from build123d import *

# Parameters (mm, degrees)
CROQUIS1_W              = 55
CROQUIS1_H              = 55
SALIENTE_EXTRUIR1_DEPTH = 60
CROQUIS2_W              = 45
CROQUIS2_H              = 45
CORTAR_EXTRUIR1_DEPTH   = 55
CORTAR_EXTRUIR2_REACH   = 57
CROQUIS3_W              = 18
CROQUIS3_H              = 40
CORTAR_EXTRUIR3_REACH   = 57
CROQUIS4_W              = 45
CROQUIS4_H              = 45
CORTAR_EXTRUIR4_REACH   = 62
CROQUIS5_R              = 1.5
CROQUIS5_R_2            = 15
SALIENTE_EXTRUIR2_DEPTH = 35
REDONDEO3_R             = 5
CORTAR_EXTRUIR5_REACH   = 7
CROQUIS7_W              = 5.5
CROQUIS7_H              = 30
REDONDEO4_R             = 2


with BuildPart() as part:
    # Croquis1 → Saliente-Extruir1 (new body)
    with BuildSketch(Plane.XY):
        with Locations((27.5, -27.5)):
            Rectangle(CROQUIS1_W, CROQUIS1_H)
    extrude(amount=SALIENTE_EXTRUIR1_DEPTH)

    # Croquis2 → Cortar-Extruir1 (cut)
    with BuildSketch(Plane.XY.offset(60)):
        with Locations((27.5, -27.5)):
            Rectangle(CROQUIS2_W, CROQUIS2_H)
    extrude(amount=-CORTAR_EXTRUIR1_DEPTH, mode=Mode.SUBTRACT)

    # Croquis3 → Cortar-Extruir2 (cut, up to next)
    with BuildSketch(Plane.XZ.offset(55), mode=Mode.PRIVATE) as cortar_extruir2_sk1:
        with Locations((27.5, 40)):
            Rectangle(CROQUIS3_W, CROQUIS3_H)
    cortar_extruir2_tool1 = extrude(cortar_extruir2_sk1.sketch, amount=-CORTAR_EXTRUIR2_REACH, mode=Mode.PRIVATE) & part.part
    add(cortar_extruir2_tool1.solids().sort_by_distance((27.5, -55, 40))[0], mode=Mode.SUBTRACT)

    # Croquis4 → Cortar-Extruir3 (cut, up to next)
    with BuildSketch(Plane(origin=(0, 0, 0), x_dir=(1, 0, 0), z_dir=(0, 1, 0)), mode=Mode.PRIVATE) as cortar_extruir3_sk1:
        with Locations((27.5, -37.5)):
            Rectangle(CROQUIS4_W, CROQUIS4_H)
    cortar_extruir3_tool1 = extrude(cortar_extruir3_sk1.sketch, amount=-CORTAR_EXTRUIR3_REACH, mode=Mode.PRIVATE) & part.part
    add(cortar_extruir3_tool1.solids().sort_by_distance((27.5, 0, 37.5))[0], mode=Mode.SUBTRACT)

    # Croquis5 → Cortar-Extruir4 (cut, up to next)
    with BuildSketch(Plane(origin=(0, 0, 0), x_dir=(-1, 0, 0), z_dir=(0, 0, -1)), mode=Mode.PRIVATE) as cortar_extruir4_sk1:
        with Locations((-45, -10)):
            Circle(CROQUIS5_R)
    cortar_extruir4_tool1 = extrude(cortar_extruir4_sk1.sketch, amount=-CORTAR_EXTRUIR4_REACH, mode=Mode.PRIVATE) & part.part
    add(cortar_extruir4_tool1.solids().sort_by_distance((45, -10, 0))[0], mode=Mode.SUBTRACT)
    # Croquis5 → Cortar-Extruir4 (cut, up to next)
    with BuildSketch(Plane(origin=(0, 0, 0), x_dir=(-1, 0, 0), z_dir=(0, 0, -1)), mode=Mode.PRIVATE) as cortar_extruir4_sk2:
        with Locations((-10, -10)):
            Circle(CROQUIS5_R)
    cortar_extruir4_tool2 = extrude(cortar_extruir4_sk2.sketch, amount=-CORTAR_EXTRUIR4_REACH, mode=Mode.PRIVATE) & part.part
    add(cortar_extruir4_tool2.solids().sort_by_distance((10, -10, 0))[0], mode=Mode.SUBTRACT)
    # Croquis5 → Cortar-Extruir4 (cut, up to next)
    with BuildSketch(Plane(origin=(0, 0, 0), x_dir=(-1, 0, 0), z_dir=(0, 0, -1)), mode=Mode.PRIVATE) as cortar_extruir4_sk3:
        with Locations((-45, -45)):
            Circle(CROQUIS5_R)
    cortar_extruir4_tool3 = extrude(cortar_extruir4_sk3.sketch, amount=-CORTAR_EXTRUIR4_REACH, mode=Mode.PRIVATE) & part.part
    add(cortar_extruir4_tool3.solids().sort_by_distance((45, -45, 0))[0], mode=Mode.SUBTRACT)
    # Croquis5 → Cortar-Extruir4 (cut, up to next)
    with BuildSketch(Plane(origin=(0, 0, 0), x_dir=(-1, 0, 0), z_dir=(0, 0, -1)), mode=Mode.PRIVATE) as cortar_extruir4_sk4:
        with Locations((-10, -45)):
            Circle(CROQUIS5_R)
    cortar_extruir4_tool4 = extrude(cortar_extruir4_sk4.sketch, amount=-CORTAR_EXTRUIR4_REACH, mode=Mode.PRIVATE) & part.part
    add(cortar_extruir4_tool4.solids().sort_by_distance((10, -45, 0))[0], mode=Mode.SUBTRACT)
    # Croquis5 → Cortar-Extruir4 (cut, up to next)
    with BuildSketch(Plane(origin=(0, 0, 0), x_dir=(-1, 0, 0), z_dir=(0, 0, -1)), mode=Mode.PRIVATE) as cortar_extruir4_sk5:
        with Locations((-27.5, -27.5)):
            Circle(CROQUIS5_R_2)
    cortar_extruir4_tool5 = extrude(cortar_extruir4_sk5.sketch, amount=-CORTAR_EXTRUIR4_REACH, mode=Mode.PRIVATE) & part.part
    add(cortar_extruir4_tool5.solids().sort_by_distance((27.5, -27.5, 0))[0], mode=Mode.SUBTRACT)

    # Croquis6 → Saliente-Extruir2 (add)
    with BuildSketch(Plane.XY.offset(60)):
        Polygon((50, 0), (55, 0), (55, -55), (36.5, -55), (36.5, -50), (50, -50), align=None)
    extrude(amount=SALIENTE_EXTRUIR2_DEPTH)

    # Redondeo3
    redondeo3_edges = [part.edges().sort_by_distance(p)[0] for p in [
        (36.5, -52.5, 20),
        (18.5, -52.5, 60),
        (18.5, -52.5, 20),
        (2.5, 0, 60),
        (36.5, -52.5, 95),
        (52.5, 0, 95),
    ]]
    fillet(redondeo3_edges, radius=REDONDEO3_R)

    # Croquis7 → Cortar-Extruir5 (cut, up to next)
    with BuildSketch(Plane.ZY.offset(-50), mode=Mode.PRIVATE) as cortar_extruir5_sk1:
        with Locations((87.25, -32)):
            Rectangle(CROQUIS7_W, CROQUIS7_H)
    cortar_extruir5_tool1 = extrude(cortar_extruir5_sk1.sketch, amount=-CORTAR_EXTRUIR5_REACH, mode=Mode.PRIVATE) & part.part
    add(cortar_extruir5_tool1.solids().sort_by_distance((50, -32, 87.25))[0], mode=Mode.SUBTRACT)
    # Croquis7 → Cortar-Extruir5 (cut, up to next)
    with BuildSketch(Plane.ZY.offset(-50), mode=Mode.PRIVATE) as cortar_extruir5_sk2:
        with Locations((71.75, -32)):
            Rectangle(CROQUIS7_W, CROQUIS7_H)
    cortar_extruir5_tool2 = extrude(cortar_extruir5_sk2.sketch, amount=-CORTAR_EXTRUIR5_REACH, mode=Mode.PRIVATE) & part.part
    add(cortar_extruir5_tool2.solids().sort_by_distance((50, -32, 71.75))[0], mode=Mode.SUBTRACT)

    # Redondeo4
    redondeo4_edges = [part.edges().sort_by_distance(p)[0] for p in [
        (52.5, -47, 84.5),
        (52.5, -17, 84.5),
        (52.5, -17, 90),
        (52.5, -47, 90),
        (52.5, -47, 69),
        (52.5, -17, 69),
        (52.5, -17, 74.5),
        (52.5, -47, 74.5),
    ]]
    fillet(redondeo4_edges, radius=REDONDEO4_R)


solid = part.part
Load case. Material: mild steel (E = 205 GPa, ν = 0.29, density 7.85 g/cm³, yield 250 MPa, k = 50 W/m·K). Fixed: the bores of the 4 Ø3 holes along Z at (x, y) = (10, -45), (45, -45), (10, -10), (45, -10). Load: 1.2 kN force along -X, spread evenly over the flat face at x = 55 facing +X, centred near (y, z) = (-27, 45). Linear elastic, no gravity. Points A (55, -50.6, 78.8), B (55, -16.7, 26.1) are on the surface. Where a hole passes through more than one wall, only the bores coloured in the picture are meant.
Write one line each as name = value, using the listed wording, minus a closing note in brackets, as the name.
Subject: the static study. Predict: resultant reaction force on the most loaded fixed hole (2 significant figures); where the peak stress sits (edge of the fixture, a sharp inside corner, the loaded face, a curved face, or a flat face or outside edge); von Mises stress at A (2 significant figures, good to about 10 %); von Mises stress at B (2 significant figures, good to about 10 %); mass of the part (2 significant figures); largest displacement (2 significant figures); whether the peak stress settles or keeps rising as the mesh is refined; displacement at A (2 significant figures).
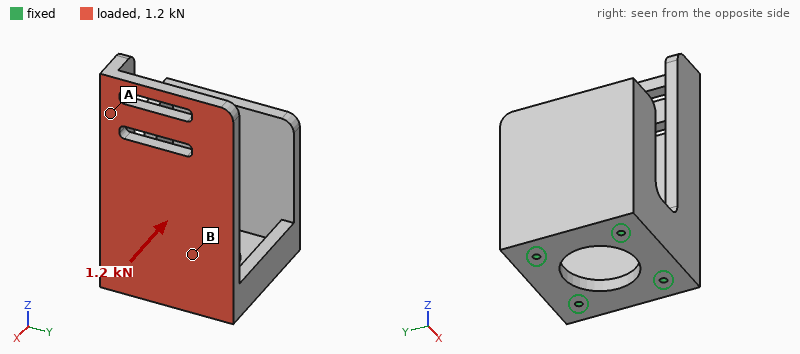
resultant reaction force on the most loaded fixed hole = 1.2 kN
where the peak stress sits = edge of the fixture
von Mises stress at A = 21 MPa
von Mises stress at B = 45 MPa
mass of the part = 490 g
largest displacement = 0.27 mm
whether the peak stress settles or keeps rising as the mesh is refined = keeps rising
displacement at A = 0.088 mm
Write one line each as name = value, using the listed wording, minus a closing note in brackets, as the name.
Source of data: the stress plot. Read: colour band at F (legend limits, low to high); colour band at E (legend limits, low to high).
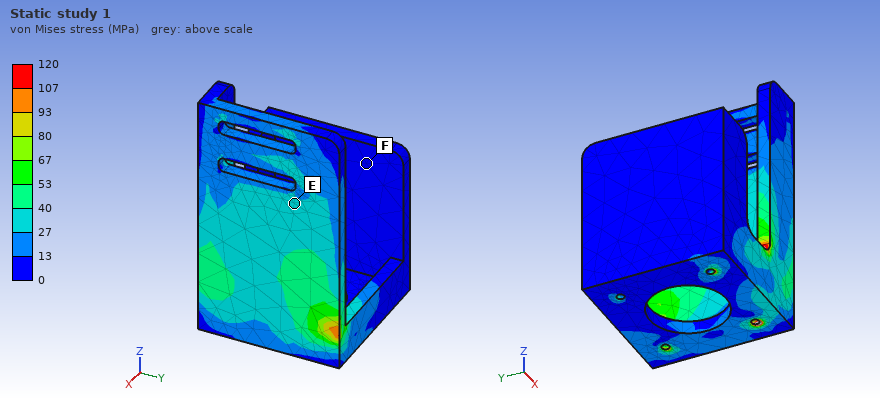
colour band at F = 0 to 13 MPa
colour band at E = 27 to 40 MPa
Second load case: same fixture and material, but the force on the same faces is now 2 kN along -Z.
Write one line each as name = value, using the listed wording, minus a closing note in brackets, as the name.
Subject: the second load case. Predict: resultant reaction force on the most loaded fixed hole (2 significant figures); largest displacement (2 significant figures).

resultant reaction force on the most loaded fixed hole = 1.3 kN
largest displacement = 54 µm
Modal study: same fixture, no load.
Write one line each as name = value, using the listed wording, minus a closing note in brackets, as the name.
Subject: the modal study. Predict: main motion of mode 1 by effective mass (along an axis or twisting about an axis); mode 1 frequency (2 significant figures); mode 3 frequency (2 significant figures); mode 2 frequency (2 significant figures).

main motion of mode 1 by effective mass = along X
mode 1 frequency = 1000 Hz
mode 3 frequency = 2200 Hz
mode 2 frequency = 2000 Hz
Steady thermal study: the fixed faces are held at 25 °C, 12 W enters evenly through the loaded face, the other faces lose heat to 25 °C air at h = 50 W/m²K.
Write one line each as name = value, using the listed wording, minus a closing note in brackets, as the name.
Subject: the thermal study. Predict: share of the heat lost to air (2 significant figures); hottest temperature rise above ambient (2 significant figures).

share of the heat lost to air = 50 %
hottest temperature rise above ambient = 17 K
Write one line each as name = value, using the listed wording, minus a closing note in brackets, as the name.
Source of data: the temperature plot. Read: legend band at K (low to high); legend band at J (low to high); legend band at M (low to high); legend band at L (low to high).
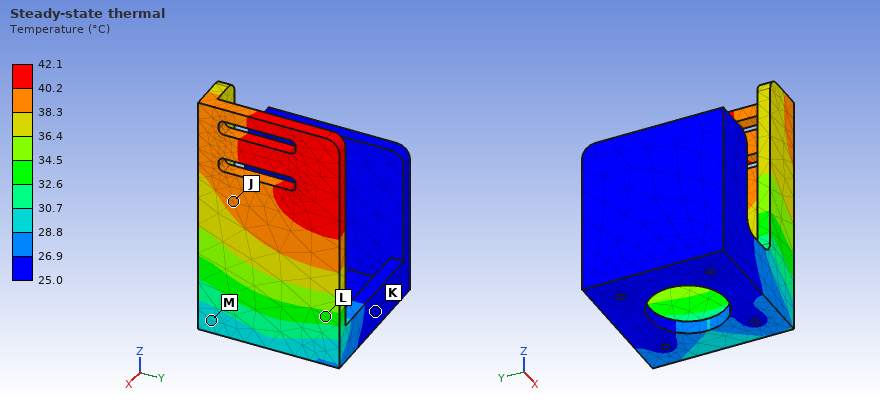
legend band at K = 25.0 to 26.9 °C
legend band at J = 38.3 to 40.2 °C
legend band at M = 28.8 to 30.7 °C
legend band at L = 32.6 to 34.5 °C
